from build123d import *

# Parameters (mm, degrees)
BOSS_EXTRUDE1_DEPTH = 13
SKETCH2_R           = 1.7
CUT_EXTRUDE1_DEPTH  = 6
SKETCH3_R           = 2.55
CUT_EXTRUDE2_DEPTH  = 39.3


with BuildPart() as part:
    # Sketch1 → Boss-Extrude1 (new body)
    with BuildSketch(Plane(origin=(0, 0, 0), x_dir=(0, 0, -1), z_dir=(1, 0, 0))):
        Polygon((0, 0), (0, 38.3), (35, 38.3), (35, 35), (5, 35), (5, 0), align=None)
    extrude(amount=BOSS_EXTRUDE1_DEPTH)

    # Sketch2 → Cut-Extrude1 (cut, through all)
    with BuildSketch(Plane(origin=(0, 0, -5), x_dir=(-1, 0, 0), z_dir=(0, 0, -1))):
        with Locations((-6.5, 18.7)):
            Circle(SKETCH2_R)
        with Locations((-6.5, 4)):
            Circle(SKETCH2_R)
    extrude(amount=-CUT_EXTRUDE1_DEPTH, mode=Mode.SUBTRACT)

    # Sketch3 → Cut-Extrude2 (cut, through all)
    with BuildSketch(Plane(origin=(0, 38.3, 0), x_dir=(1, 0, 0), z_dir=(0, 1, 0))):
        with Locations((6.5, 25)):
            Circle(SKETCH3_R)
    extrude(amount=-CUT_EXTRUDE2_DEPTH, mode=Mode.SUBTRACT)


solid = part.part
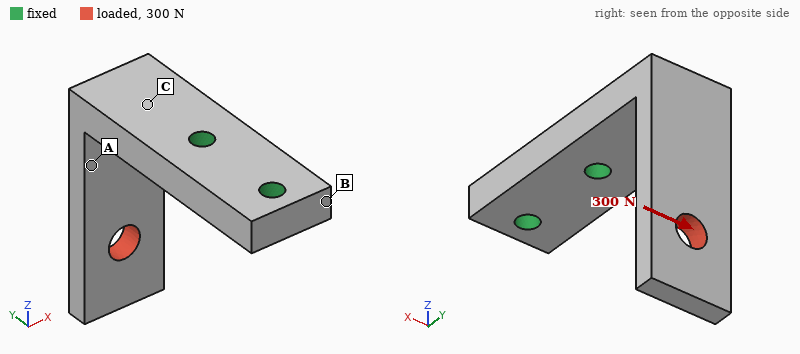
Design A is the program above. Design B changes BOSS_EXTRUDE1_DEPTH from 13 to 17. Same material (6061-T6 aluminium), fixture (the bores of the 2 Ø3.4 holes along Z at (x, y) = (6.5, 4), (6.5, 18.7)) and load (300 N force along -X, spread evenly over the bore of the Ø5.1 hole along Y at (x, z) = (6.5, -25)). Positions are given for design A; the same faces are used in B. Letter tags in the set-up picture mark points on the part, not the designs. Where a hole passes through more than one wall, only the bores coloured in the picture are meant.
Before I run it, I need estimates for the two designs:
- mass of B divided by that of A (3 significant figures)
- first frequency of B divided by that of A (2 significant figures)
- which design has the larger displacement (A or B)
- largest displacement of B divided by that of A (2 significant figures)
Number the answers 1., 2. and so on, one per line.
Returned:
1. 1.32
2. 0.99
3. A
4. 0.72
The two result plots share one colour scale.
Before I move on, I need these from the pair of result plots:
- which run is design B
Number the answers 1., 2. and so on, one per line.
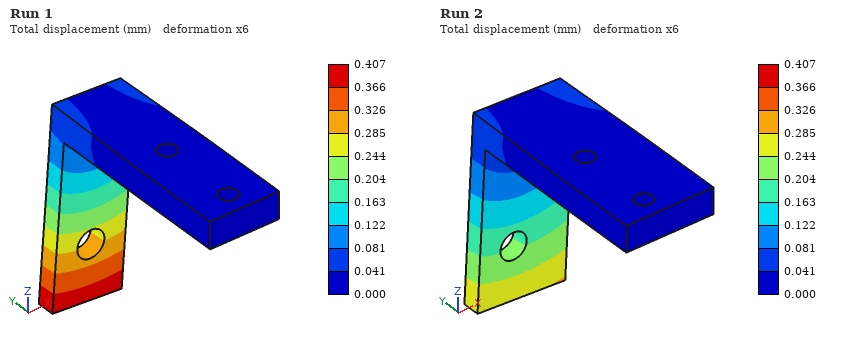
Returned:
1. Run 2
